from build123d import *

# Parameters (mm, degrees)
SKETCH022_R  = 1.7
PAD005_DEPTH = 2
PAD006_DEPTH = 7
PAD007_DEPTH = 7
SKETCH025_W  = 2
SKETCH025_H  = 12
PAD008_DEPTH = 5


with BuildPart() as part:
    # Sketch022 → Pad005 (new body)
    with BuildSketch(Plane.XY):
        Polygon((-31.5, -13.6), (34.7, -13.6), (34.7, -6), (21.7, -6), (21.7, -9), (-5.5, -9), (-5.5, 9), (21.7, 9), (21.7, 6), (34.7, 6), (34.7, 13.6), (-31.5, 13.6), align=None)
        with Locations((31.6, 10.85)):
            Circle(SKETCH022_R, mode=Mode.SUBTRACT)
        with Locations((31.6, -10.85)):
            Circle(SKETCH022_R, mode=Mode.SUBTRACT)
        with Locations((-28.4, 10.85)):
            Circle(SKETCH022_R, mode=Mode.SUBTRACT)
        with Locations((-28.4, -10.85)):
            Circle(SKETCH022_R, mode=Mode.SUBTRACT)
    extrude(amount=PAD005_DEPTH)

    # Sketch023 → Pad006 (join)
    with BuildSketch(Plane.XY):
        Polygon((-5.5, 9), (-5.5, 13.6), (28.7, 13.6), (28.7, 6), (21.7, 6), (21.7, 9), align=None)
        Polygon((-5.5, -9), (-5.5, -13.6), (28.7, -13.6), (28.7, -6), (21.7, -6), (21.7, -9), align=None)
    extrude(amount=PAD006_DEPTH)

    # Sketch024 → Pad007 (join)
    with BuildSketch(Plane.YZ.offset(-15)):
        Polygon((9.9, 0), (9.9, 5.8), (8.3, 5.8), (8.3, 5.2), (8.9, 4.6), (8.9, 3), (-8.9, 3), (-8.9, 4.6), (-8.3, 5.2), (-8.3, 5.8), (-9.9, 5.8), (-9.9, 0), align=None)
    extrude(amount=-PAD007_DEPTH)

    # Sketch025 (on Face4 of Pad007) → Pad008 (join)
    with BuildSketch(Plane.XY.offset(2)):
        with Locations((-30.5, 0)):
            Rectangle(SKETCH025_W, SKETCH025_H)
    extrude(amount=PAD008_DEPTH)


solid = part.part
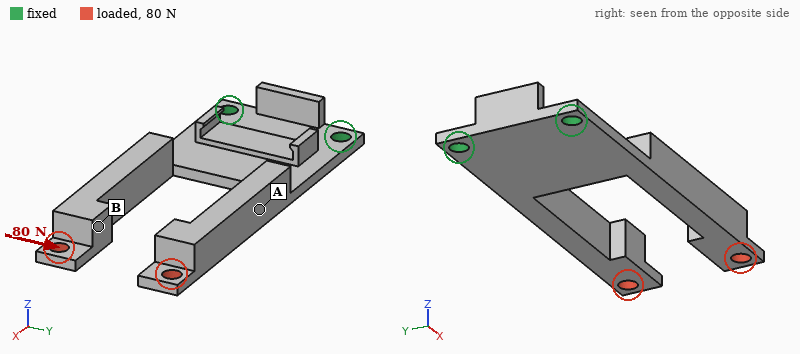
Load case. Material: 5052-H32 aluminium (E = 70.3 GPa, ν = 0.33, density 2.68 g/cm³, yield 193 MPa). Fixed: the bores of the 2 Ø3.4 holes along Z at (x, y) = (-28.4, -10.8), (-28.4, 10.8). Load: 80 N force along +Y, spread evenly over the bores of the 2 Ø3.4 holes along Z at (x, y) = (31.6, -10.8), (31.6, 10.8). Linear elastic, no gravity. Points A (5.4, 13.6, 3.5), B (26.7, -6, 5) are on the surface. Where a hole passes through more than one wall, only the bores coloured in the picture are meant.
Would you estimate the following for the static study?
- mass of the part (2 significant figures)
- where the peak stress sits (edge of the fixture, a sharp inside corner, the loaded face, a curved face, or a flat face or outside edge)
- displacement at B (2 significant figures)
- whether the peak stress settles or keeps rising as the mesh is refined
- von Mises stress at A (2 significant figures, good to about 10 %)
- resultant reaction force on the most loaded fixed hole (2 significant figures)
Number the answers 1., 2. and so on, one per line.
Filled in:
1. 12 g
2. a sharp inside corner
3. 0.34 mm
4. keeps rising
5. 43 MPa
6. 220 N
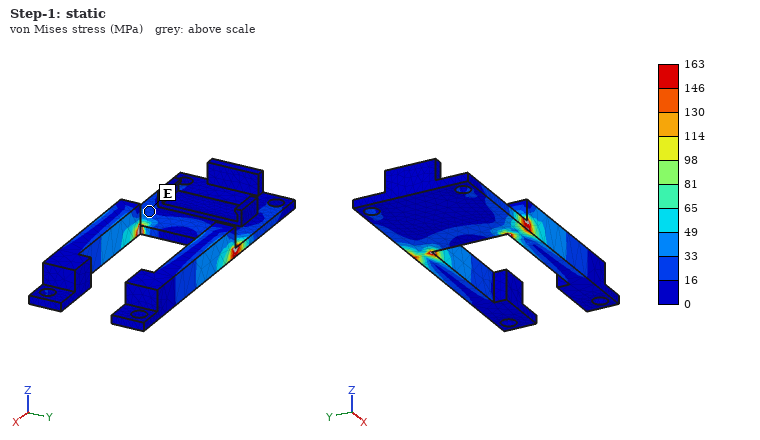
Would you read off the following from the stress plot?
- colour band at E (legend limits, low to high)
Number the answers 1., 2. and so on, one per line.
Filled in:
1. 16 to 33 MPa
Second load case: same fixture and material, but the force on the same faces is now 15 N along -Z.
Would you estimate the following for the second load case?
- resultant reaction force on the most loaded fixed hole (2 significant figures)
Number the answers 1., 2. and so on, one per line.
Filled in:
1. 8.9 N
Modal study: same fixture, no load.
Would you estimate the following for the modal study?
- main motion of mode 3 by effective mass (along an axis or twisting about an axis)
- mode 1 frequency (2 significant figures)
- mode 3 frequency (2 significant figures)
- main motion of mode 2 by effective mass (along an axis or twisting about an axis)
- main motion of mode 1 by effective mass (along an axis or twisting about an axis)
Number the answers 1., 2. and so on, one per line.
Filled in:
1. along Y
2. 410 Hz
3. 1500 Hz
4. twisting about X
5. along Z
